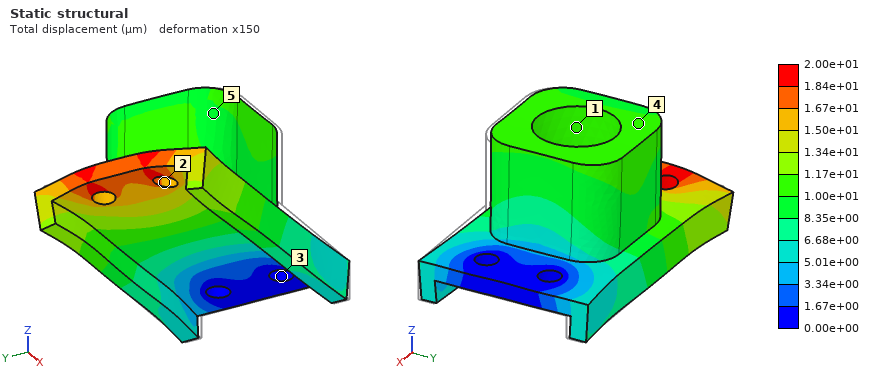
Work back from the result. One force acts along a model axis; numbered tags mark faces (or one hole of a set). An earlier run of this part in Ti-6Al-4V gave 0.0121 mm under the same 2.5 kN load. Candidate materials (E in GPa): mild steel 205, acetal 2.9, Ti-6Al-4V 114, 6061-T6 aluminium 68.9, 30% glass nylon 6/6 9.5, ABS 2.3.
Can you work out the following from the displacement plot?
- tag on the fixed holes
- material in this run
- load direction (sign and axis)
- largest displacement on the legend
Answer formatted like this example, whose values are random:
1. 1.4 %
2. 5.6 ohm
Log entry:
1. 3
2. 6061-T6 aluminium
3. -X
4. 2.00e+01 µm
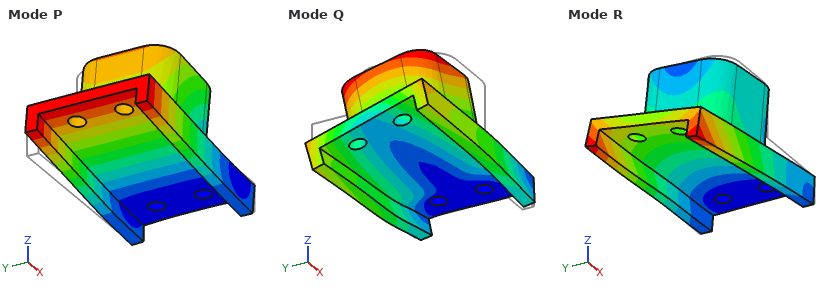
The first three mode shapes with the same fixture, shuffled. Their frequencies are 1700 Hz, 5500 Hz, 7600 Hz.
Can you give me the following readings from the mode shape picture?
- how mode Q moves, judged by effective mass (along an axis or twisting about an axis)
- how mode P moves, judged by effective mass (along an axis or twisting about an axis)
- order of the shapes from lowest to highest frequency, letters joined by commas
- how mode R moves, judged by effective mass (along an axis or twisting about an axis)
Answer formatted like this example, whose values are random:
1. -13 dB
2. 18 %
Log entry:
1. along Y
2. along Z
3. P, Q, R
4. along Y
